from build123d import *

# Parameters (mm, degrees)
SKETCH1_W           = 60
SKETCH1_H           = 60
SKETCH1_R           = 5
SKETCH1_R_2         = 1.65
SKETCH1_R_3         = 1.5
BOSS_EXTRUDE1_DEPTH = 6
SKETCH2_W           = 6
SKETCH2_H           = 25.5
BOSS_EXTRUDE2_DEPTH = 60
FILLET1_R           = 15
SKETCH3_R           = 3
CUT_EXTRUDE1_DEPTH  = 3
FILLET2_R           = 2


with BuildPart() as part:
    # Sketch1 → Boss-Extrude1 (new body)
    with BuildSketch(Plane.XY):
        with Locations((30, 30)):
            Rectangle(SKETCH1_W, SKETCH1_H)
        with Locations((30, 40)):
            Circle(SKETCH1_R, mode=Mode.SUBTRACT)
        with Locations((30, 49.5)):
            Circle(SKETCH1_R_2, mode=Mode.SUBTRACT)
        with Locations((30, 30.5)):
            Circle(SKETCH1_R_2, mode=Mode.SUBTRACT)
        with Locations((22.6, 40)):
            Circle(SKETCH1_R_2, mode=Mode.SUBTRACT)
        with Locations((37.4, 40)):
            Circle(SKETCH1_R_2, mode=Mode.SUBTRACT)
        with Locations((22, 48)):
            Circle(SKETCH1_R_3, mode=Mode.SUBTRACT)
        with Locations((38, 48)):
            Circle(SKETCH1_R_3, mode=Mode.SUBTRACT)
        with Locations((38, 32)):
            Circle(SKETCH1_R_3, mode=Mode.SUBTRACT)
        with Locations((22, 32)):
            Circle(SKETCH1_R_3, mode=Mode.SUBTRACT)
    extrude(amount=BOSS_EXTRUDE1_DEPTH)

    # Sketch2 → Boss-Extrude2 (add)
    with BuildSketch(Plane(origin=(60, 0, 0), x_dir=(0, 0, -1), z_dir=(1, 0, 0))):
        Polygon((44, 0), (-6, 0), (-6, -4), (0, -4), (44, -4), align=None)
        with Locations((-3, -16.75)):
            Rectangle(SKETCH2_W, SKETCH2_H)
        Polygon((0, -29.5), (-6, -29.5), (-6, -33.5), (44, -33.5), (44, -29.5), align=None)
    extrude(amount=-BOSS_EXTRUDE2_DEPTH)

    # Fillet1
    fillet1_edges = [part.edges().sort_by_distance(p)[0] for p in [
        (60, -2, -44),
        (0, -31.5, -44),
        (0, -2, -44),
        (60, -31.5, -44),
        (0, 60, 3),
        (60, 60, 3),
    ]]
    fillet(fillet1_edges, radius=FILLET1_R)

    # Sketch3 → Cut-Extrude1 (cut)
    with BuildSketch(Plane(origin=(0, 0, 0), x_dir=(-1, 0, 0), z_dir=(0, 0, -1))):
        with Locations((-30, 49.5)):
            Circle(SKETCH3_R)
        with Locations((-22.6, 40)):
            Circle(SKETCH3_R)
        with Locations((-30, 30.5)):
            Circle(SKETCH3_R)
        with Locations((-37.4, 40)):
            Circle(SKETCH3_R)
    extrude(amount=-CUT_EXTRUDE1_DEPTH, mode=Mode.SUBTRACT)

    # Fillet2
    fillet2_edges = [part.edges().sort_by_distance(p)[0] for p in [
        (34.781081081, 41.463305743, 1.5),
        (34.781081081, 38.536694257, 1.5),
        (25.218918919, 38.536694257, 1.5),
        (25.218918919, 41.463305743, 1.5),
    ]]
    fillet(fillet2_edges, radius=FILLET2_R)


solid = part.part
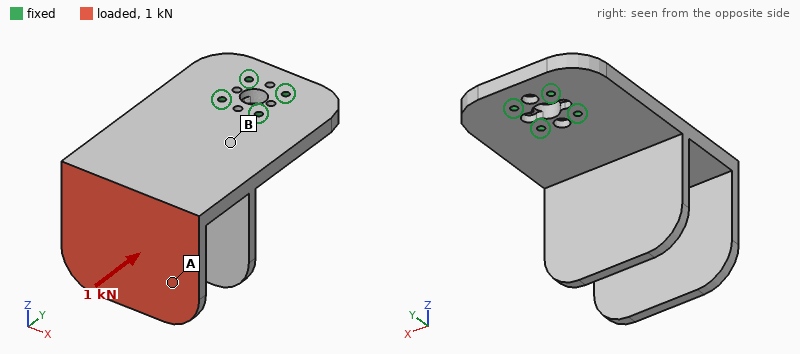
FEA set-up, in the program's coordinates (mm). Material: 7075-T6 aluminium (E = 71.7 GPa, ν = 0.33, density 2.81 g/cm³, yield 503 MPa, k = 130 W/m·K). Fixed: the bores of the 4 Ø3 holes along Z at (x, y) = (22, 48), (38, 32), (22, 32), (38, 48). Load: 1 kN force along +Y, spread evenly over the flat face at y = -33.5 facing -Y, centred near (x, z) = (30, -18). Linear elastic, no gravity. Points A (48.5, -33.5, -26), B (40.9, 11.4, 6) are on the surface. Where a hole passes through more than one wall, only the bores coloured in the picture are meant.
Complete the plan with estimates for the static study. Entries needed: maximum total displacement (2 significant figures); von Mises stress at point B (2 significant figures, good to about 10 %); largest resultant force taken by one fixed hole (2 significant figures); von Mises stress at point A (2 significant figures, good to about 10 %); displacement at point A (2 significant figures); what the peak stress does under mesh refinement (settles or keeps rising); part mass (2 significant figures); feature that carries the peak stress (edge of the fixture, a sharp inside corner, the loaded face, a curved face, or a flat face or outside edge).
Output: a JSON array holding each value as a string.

["1.3 mm", "50 MPa", "500 N", "18 MPa", "0.92 mm", "keeps rising", "150 g", "edge of the fixture"]
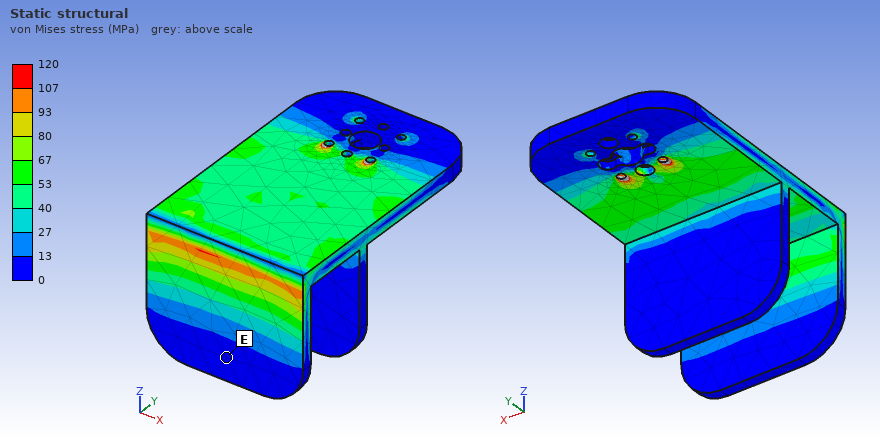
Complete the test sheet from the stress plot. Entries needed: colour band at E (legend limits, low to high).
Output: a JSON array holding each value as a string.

["0 to 13 MPa"]
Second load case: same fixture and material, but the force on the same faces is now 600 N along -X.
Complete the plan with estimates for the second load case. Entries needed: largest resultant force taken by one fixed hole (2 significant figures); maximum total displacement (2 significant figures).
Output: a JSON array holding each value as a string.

["1.2 kN", "0.31 mm"]
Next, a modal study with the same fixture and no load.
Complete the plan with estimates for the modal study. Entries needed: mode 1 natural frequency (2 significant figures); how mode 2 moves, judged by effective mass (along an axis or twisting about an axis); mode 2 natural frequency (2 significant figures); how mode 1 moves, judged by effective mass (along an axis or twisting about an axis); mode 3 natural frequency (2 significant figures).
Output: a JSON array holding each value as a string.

["550 Hz", "along X", "1100 Hz", "along Z", "1400 Hz"]
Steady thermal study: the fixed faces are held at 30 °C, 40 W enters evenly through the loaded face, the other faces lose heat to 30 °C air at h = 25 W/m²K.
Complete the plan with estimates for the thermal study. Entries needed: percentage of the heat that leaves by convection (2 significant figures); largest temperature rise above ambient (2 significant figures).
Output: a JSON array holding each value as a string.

["32 %", "66 K"]
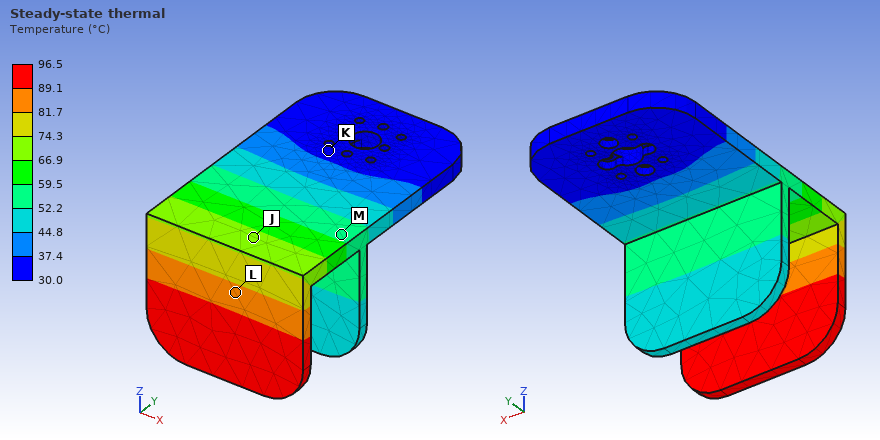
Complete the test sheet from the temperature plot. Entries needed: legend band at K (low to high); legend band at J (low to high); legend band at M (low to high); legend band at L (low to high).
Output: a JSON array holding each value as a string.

["30.0 to 37.4 °C", "66.9 to 74.3 °C", "52.2 to 59.5 °C", "81.7 to 89.1 °C"]
